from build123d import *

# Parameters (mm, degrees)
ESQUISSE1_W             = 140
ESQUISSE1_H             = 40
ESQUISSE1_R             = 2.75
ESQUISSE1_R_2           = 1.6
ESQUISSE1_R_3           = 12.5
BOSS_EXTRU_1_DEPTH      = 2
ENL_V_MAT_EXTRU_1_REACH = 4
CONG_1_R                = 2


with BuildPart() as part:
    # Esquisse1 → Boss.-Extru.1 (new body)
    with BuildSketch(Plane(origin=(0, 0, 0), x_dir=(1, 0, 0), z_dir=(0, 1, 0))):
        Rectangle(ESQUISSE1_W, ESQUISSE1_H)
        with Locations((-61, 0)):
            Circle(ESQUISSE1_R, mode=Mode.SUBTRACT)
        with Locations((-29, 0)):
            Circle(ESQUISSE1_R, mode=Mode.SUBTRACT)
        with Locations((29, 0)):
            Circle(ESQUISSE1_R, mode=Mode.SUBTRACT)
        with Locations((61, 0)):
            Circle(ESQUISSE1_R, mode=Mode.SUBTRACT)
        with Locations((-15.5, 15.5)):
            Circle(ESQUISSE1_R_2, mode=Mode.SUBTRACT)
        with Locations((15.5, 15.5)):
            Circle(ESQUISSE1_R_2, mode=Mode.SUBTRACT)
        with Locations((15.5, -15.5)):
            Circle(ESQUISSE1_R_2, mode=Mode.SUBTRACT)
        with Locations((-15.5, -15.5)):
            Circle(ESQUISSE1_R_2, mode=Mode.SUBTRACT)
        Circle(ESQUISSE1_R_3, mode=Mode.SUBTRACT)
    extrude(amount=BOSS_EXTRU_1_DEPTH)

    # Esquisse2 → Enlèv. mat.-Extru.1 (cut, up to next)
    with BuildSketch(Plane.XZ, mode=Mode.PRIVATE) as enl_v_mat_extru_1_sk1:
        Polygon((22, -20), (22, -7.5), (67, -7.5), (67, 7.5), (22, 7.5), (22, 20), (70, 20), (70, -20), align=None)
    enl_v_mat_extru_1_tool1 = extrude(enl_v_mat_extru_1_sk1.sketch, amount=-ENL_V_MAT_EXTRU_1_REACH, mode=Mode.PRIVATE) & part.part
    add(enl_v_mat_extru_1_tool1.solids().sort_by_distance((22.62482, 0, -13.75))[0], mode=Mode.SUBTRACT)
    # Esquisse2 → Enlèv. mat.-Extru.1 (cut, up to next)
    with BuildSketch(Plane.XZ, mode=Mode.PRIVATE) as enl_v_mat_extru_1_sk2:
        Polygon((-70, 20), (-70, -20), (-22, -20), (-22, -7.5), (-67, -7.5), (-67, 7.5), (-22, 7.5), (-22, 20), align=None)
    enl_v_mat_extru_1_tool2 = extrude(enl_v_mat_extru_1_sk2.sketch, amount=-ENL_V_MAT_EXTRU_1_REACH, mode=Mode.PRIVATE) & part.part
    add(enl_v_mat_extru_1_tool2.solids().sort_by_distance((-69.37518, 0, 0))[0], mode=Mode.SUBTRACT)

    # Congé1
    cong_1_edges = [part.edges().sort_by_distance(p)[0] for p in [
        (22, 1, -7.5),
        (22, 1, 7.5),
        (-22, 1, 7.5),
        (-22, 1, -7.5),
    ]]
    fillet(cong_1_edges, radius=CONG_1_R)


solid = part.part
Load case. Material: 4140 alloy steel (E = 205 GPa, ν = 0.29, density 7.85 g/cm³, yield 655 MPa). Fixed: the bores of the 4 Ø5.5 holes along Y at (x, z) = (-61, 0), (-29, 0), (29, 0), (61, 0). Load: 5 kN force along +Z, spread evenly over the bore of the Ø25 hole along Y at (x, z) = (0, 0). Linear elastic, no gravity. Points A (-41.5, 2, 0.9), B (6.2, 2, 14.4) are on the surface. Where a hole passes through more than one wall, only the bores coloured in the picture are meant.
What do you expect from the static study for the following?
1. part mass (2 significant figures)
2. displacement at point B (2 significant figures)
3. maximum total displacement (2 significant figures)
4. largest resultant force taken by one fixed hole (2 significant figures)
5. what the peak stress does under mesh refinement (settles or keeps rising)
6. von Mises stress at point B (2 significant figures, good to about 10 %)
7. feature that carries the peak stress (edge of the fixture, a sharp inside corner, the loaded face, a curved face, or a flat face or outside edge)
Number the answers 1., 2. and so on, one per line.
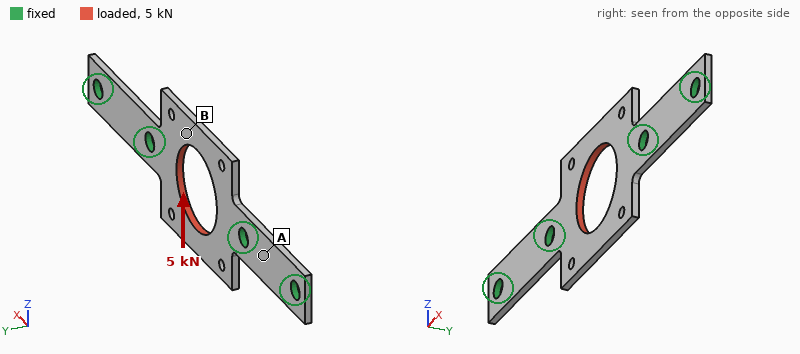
1. 39 g
2. 21 µm
3. 23 µm
4. 2.6 kN
5. keeps rising
6. 79 MPa
7. edge of the fixture
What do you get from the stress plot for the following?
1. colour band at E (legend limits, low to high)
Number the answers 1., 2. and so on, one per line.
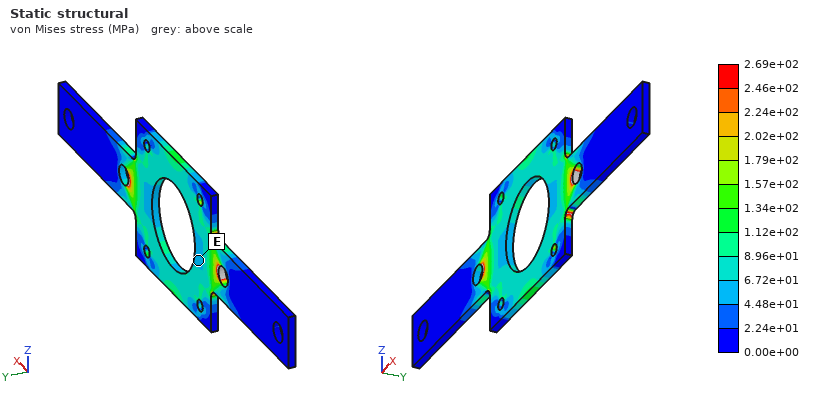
1. 4.48e+01 to 6.72e+01 MPa
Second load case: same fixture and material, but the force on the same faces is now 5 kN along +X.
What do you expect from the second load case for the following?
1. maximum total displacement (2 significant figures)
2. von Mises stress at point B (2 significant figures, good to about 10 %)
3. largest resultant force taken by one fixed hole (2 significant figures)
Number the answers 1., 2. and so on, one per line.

1. 12 µm
2. 27 MPa
3. 2.4 kN
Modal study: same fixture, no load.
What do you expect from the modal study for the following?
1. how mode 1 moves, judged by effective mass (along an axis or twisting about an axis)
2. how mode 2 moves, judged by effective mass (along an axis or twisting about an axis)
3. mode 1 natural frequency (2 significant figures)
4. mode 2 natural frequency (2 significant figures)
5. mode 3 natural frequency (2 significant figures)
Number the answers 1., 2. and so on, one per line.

1. twisting about X
2. along Y
3. 2200 Hz
4. 2500 Hz
5. 5100 Hz
